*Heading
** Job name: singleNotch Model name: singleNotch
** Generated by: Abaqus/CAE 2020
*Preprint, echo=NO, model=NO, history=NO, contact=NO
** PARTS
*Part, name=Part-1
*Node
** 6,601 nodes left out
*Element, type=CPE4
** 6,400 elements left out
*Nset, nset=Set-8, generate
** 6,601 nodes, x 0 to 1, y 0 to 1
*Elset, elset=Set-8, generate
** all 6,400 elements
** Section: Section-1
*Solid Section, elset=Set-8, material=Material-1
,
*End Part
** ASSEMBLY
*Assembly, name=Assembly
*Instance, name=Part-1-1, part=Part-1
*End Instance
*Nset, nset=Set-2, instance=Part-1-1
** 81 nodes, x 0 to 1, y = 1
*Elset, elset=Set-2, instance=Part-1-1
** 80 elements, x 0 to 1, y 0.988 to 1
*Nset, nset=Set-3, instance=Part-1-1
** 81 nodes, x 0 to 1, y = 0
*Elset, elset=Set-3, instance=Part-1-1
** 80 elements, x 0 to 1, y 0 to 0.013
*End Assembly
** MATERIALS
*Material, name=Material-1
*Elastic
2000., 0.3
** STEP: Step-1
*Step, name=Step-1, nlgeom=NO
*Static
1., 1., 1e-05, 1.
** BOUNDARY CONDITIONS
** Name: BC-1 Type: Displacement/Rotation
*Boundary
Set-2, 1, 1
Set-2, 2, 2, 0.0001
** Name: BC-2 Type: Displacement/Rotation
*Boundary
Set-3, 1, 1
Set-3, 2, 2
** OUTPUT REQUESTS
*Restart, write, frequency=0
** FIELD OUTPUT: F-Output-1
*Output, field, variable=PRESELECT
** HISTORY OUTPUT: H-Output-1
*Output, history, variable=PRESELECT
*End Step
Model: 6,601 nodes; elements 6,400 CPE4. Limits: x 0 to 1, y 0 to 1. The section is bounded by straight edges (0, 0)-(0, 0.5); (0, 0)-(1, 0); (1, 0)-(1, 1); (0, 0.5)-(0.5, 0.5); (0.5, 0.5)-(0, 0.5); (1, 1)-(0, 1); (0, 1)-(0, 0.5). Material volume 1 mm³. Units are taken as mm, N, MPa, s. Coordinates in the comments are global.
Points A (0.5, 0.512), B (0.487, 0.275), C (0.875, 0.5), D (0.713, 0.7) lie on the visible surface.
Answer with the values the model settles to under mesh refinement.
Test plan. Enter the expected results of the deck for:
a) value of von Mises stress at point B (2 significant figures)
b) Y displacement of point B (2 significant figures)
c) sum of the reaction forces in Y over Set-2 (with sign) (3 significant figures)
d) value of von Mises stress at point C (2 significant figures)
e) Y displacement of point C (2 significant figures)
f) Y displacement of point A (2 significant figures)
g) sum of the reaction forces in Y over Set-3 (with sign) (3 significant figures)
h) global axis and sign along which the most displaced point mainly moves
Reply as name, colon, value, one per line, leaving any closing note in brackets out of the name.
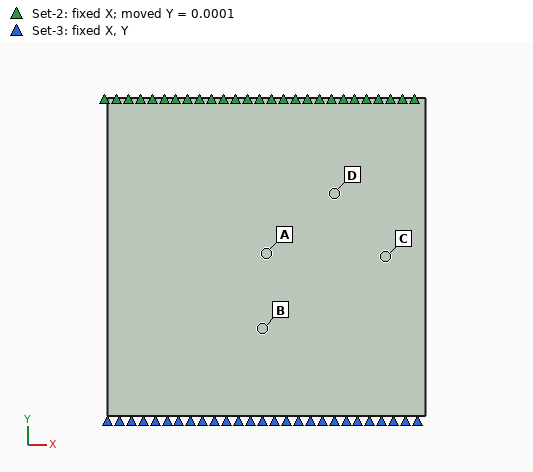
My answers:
value of von Mises stress at point B: 0.16 MPa
Y displacement of point B: 1.8e-05 mm
sum of the reaction forces in Y over Set-2 (with sign): 0.135 N
value of von Mises stress at point C: 0.18 MPa
Y displacement of point C: 5.0e-05 mm
Y displacement of point A: 5.6e-05 mm
sum of the reaction forces in Y over Set-3 (with sign): -0.135 N
global axis and sign along which the most displaced point mainly moves: +Y
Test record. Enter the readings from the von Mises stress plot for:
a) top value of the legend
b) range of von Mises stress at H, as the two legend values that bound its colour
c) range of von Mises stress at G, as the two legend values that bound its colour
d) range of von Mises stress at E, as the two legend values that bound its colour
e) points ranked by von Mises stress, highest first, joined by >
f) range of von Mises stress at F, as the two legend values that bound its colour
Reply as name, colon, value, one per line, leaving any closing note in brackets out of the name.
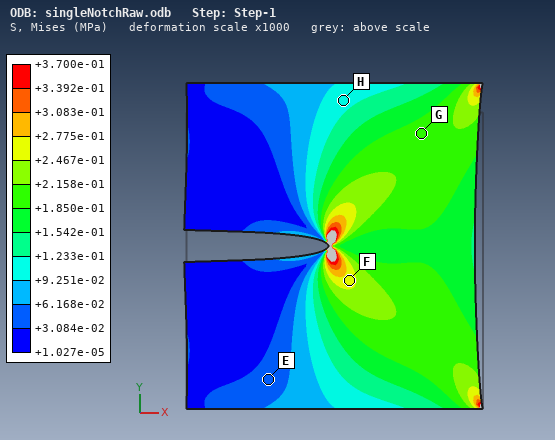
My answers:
top value of the legend: +3.700e-01 MPa
range of von Mises stress at H, as the two legend values that bound its colour: +9.251e-02 to +1.233e-01 MPa
range of von Mises stress at G, as the two legend values that bound its colour: +1.850e-01 to +2.158e-01 MPa
range of von Mises stress at E, as the two legend values that bound its colour: +3.084e-02 to +6.168e-02 MPa
points ranked by von Mises stress, highest first, joined by >: F > G > H > E
range of von Mises stress at F, as the two legend values that bound its colour: +2.467e-01 to +2.775e-01 MPa
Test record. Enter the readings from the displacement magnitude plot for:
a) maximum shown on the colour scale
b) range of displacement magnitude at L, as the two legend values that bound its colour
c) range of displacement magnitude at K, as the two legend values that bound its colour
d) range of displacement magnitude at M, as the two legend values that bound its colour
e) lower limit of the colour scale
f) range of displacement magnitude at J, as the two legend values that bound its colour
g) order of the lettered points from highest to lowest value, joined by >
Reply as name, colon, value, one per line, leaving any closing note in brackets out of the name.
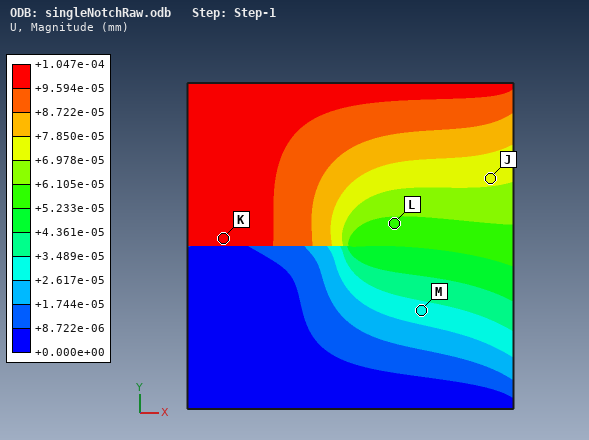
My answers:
maximum shown on the colour scale: +1.047e-04 mm
range of displacement magnitude at L, as the two legend values that bound its colour: +5.233e-05 to +6.105e-05 mm
range of displacement magnitude at K, as the two legend values that bound its colour: +9.594e-05 to +1.047e-04 mm
range of displacement magnitude at M, as the two legend values that bound its colour: +2.617e-05 to +3.489e-05 mm
lower limit of the colour scale: +0.000e+00 mm
range of displacement magnitude at J, as the two legend values that bound its colour: +6.978e-05 to +7.850e-05 mm
order of the lettered points from highest to lowest value, joined by >: K > J > L > M
